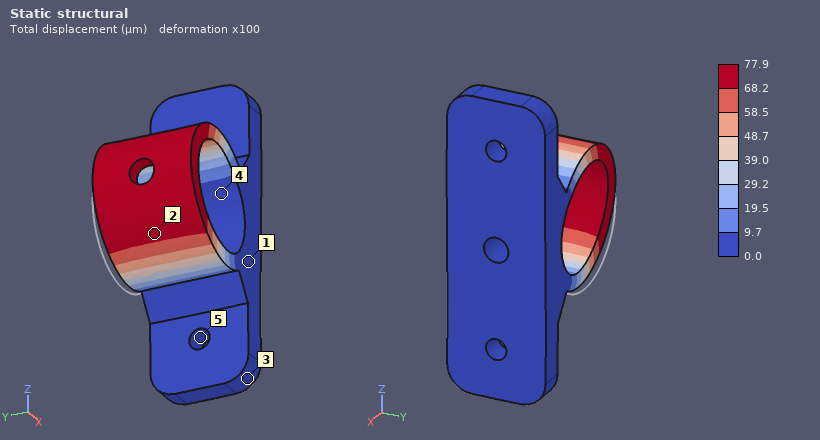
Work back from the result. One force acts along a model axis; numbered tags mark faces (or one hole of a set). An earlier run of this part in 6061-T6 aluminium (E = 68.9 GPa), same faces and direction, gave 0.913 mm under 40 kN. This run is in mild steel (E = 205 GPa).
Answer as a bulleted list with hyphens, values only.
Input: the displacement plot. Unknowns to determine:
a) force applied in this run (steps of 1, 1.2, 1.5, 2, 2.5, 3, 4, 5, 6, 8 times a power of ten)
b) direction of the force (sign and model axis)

- 10 kN
- +Z
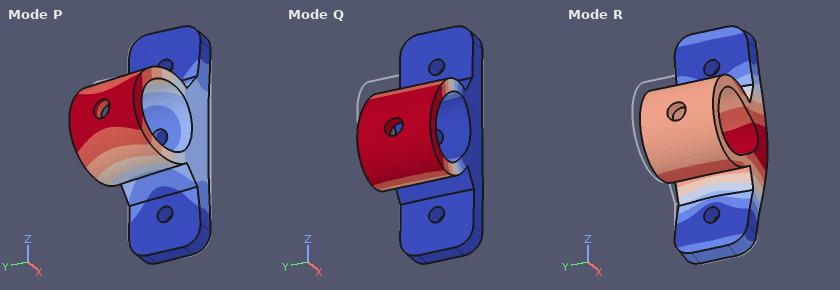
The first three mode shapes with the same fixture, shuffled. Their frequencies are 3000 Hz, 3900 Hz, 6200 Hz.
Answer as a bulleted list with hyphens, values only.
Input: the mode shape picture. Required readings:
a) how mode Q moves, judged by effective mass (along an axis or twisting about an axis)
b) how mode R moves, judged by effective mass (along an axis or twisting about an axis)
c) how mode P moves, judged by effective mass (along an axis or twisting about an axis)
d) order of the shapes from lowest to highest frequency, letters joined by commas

- along Z
- along X
- along Y
- P, Q, R
